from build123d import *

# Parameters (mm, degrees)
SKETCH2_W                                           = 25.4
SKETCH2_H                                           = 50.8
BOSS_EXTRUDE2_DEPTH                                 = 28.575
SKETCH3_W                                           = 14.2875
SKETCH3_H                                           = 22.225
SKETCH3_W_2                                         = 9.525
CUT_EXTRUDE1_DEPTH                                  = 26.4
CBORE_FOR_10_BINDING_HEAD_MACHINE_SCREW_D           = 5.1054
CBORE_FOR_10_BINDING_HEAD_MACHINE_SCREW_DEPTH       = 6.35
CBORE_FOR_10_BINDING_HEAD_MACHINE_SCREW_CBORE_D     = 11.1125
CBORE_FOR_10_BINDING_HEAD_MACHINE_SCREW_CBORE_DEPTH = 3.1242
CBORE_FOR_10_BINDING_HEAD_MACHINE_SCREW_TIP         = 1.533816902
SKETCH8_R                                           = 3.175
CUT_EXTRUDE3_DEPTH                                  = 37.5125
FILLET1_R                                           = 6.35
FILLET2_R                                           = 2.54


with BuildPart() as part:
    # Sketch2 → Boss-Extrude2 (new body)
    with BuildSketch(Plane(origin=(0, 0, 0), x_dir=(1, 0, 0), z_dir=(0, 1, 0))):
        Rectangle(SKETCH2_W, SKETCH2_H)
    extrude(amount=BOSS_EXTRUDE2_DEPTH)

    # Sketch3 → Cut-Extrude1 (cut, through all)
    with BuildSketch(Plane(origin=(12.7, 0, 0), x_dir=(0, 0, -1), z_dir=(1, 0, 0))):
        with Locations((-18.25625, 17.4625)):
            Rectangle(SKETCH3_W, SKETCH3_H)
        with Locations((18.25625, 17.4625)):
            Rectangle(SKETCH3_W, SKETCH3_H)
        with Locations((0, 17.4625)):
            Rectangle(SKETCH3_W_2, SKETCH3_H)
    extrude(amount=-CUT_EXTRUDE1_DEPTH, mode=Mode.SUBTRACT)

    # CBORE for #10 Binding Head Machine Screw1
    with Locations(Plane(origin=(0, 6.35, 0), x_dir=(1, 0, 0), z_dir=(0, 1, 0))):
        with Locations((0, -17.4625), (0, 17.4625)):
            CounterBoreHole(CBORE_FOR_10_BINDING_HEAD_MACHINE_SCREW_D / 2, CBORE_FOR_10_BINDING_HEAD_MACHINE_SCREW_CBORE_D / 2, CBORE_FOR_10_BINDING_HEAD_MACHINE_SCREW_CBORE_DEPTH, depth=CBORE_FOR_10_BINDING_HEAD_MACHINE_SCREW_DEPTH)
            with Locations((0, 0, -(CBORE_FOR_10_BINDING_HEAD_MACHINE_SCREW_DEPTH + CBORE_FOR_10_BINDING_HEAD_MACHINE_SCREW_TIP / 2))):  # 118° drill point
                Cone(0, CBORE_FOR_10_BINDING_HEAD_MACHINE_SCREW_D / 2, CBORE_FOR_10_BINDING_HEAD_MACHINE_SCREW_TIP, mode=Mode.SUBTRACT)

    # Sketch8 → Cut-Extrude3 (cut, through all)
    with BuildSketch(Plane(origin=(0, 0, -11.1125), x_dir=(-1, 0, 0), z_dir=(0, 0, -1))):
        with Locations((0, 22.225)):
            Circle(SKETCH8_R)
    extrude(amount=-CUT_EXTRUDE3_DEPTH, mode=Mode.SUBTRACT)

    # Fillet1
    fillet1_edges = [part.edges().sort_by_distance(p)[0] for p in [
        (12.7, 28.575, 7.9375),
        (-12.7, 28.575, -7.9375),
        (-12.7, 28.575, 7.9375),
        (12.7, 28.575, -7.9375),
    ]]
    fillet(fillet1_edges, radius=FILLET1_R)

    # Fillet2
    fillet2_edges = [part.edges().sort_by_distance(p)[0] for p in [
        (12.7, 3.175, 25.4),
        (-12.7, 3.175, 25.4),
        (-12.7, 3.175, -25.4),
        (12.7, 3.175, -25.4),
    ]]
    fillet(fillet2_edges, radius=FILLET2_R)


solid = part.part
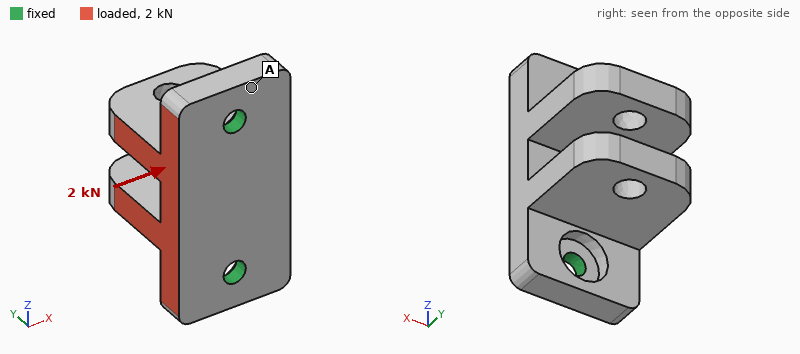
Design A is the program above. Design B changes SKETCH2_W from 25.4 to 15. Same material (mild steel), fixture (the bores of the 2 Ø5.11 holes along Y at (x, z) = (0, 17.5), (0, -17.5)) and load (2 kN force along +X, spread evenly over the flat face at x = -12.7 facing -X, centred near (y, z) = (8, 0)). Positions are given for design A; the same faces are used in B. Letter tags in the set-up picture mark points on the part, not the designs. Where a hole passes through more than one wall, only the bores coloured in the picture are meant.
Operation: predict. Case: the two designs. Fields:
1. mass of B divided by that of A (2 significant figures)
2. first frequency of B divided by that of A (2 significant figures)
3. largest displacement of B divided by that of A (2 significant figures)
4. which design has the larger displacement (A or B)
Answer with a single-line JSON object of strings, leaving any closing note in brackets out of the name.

{"mass of B divided by that of A": "0.55", "first frequency of B divided by that of A": "1.3", "largest displacement of B divided by that of A": "1.4", "which design has the larger displacement": "B"}
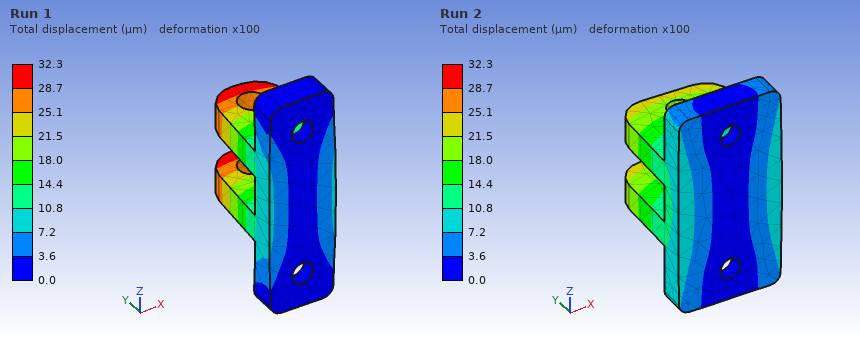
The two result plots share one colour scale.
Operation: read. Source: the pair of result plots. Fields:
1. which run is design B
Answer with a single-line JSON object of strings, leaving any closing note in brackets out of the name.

{"which run is design B": "Run 1"}
